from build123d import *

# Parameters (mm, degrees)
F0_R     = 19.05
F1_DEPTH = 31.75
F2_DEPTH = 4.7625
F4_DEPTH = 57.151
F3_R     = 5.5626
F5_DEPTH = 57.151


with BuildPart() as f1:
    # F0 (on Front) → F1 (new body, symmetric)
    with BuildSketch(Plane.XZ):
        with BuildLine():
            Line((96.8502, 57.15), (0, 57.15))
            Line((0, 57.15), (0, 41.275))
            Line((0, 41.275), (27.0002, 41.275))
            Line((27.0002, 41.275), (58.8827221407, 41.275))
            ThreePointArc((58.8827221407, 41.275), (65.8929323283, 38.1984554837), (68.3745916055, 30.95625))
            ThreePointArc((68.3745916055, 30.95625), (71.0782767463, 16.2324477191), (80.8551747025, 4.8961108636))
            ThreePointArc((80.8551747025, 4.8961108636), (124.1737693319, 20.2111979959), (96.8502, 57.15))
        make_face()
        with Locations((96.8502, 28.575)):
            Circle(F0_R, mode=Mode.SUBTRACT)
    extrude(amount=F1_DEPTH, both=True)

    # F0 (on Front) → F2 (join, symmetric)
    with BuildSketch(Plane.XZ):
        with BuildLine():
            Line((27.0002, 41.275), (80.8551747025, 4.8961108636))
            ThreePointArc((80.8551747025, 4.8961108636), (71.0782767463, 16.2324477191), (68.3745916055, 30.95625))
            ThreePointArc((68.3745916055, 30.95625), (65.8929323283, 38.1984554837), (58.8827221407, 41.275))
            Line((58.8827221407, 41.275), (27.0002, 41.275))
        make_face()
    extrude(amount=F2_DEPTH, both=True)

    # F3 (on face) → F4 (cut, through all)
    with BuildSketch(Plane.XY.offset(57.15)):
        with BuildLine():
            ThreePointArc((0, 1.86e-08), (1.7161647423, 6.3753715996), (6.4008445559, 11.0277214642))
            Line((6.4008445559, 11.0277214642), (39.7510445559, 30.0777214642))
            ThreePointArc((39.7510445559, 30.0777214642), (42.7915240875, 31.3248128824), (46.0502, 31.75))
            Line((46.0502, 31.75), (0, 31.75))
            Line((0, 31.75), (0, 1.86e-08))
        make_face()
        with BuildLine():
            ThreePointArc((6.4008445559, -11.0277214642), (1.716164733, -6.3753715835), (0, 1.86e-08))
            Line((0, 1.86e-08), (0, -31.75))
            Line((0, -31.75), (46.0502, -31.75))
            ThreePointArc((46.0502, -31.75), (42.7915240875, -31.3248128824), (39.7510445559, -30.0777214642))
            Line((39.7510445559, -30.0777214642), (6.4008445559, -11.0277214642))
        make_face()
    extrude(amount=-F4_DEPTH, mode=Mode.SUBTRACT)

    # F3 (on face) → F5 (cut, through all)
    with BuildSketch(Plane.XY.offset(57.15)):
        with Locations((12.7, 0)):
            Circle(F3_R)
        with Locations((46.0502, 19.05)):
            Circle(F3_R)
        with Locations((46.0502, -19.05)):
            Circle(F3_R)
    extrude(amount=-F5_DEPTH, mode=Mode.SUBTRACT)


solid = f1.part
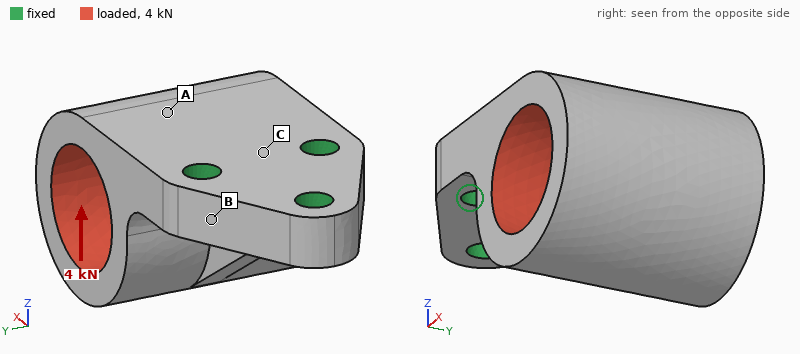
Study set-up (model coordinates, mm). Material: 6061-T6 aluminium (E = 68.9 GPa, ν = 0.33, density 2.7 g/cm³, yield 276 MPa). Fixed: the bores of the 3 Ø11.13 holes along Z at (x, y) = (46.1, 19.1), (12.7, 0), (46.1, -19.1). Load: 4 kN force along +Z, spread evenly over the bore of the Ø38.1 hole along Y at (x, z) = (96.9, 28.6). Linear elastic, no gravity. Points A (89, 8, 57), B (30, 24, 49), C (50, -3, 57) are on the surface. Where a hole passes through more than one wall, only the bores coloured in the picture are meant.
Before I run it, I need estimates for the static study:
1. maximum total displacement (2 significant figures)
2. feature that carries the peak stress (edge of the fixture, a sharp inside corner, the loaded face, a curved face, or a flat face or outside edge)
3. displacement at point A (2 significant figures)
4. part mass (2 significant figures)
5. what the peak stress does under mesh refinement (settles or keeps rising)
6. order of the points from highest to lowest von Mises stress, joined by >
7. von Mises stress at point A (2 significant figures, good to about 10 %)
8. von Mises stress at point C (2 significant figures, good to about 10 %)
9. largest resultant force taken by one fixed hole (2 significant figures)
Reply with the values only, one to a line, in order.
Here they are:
0.13 mm
edge of the fixture
0.056 mm
420 g
keeps rising
C > A > B
14 MPa
25 MPa
2.9 kN
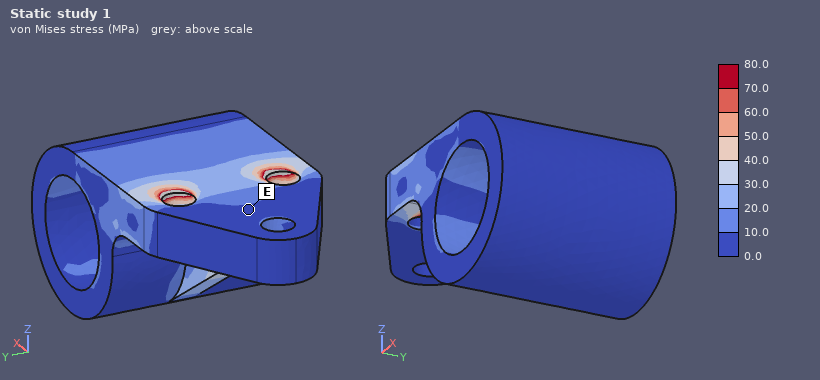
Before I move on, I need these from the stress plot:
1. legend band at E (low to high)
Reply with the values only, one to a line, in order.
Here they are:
0.0 to 10.0 MPa
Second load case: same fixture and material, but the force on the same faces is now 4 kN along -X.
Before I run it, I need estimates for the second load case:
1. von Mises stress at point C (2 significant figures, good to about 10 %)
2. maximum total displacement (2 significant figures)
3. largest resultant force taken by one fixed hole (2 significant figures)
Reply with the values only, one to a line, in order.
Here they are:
9.1 MPa
62 µm
1.6 kN
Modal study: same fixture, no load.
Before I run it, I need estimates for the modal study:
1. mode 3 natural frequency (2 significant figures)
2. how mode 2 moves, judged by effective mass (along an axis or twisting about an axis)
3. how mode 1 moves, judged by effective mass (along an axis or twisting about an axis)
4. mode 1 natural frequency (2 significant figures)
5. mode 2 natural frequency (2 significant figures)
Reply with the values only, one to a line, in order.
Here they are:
5900 Hz
along Y
along Z
1900 Hz
3600 Hz
